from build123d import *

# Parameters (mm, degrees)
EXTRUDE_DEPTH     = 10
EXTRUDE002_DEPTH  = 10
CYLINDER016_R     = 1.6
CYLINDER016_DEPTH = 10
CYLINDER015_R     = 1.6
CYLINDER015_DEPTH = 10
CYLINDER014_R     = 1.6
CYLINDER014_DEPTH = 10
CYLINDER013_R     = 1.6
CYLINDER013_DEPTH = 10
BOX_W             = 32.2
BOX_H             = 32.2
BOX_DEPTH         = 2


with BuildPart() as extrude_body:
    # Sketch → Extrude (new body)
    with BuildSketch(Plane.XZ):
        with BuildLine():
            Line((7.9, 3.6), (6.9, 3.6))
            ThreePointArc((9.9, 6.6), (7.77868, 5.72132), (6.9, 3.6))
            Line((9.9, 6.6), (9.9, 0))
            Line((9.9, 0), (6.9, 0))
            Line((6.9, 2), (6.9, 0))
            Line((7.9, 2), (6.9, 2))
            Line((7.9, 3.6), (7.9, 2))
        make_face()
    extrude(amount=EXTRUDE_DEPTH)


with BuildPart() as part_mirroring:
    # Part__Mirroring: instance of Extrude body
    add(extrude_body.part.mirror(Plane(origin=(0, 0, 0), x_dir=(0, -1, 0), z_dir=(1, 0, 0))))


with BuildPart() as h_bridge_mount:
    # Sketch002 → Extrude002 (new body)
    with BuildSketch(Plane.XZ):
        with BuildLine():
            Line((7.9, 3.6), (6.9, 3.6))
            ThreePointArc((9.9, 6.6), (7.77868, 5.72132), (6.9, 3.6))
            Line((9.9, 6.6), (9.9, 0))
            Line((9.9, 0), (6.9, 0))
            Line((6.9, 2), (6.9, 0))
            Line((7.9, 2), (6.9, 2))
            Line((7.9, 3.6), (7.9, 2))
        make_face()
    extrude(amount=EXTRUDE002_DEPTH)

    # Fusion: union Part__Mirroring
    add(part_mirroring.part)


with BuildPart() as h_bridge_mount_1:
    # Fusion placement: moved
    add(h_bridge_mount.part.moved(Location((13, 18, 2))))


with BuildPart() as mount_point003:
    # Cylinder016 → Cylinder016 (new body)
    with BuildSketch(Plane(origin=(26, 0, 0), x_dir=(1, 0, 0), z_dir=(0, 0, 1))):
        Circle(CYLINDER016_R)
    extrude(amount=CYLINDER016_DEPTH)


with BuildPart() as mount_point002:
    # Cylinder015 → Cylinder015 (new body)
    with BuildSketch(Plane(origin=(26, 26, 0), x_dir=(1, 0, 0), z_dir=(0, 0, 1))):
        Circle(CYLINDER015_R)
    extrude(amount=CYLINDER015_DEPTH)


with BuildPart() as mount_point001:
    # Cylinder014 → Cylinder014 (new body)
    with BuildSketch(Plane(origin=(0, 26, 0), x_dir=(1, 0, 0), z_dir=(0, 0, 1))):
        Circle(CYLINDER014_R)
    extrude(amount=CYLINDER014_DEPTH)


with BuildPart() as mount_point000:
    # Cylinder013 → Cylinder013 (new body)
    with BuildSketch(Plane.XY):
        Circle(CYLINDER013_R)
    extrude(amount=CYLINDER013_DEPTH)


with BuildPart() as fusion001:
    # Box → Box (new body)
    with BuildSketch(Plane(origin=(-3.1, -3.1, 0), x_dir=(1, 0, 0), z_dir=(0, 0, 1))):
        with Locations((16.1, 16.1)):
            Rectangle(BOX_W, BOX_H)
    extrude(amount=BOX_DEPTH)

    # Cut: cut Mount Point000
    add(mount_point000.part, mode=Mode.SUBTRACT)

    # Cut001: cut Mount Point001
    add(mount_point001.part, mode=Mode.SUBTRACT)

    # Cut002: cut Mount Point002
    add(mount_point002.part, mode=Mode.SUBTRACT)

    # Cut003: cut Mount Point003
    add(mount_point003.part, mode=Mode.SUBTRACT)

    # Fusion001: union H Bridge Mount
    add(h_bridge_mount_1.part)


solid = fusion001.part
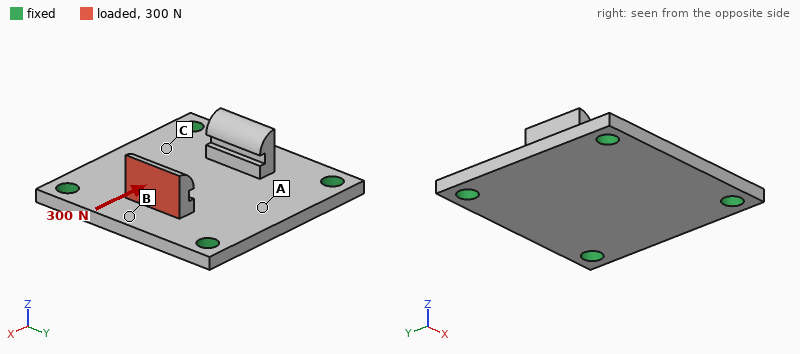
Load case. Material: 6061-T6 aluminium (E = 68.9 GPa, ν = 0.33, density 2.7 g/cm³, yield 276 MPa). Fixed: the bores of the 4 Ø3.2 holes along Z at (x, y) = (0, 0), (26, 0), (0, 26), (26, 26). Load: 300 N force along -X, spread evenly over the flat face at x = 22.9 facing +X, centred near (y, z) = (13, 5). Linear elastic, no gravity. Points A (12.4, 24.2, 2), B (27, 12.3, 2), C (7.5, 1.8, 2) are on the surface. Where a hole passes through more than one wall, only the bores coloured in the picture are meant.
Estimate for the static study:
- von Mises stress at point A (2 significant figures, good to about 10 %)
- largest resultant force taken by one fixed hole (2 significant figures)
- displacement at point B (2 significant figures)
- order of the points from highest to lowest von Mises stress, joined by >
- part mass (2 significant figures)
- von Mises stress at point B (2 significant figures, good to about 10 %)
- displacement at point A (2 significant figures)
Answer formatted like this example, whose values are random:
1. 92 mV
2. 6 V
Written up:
1. 11 MPa
2. 98 N
3. 14 µm
4. B > A > C
5. 6.3 g
6. 20 MPa
7. 7.0 µm
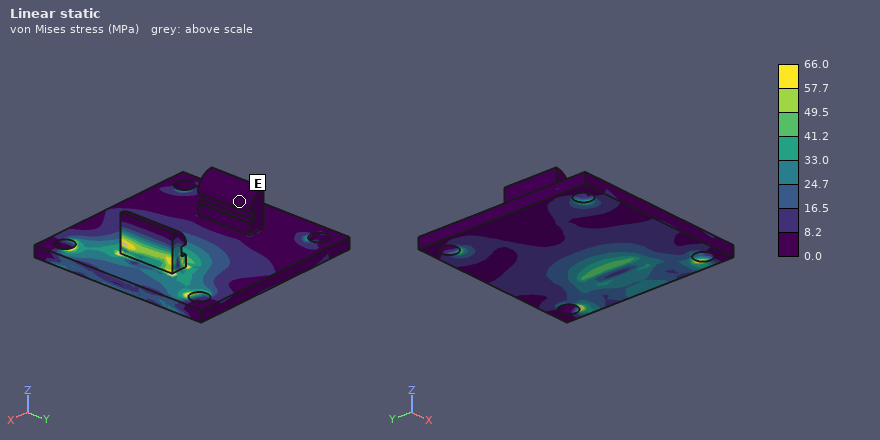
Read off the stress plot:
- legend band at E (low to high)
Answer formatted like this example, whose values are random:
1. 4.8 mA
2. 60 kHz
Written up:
1. 0.0 to 8.2 MPa
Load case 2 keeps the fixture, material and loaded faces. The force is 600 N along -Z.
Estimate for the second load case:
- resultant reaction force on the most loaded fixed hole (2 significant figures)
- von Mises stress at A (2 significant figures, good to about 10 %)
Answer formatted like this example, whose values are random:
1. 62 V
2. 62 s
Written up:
1. 280 N
2. 20 MPa
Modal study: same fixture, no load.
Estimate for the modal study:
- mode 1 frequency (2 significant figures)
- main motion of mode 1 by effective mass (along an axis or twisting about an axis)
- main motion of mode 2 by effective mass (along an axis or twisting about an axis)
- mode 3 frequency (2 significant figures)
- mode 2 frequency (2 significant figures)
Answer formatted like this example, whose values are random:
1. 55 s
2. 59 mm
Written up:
1. 11 kHz
2. along Z
3. twisting about Y
4. 19 kHz
5. 17 kHz
